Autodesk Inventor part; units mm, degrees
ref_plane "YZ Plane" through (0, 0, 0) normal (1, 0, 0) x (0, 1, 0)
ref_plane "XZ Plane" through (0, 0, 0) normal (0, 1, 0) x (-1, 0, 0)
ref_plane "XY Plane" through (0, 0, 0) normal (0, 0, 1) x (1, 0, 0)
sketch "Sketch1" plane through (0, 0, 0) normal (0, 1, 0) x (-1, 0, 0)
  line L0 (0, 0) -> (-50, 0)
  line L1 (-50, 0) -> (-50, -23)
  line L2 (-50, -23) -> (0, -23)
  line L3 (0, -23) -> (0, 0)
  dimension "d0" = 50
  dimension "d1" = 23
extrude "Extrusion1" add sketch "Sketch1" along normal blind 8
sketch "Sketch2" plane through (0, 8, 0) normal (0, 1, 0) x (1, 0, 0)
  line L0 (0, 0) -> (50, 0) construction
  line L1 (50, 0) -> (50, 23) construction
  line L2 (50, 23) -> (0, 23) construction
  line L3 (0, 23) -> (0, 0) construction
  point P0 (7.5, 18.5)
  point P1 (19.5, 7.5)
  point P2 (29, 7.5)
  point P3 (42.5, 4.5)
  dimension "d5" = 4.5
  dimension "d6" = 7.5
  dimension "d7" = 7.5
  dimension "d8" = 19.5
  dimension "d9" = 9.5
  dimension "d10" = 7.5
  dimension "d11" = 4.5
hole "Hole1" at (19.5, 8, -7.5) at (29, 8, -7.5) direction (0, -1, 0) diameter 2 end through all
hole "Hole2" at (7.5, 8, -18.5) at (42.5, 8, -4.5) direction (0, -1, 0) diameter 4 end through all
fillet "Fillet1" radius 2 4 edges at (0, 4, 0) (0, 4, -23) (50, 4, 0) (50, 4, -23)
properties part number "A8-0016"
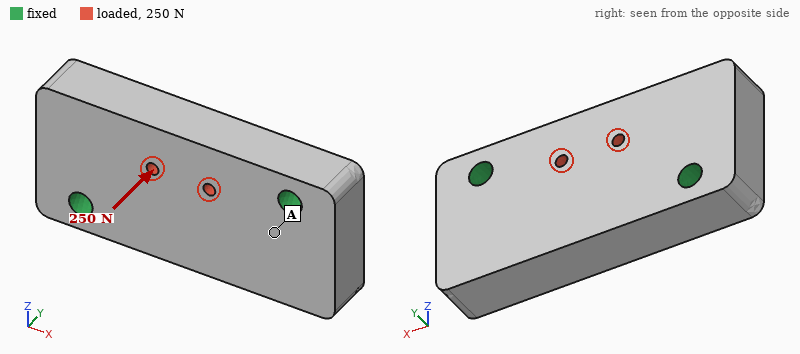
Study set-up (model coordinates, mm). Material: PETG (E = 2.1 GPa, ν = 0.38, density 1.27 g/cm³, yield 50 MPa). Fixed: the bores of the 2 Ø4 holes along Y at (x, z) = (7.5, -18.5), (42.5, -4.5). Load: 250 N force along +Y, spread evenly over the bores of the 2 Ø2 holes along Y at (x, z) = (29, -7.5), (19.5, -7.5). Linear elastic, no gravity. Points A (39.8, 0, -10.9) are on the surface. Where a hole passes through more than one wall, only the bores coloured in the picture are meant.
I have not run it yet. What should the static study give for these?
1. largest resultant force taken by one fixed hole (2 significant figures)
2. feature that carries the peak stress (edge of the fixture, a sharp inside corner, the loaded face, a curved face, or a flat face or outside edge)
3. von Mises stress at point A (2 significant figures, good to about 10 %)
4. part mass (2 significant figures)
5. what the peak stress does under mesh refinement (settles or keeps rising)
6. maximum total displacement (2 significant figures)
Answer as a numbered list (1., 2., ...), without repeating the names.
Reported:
1. 130 N
2. edge of the fixture
3. 1.8 MPa
4. 11 g
5. keeps rising
6. 0.10 mm
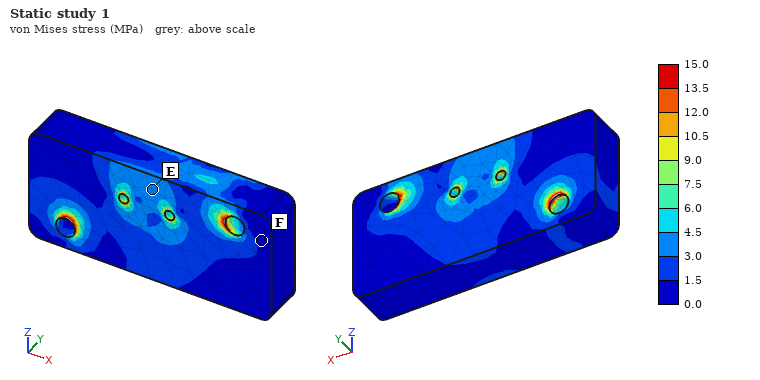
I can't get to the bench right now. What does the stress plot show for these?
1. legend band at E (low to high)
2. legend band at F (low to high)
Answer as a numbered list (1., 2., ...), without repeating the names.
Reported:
1. 3.0 to 4.5 MPa
2. 0.0 to 1.5 MPa
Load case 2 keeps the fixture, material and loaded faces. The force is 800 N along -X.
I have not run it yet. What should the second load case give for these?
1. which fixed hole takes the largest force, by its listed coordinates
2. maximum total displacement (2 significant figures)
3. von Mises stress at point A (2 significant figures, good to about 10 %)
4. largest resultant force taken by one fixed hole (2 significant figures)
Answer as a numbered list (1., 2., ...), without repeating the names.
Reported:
1. (42.5, -4.5)
2. 56 µm
3. 2.3 MPa
4. 450 N
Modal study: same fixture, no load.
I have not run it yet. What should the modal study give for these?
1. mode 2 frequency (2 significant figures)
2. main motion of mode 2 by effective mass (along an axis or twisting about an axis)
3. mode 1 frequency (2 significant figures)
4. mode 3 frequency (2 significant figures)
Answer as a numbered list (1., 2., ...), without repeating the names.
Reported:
1. 4400 Hz
2. along Y
3. 3900 Hz
4. 6300 Hz
